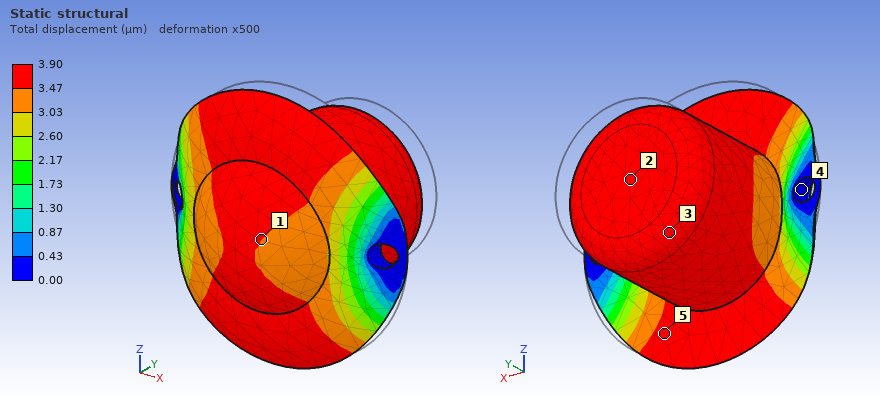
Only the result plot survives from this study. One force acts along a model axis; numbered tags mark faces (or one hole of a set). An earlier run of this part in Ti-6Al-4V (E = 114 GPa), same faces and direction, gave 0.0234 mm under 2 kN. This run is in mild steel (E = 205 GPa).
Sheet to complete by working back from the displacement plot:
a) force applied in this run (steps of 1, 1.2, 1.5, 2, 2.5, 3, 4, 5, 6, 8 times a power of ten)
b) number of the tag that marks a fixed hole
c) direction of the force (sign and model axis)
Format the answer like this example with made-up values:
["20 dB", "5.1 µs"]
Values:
["600 N", "4", "-Y"]
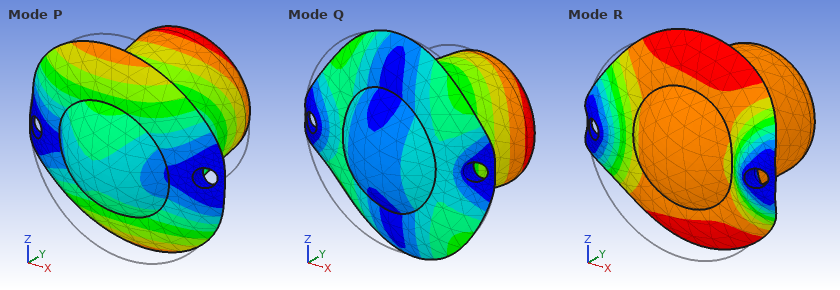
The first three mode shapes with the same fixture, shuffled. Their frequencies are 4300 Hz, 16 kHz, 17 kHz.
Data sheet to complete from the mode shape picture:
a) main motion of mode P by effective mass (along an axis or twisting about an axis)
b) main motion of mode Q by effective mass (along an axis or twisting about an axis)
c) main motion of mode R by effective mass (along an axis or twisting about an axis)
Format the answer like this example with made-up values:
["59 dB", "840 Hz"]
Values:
["along Z", "along X", "along Y"]
